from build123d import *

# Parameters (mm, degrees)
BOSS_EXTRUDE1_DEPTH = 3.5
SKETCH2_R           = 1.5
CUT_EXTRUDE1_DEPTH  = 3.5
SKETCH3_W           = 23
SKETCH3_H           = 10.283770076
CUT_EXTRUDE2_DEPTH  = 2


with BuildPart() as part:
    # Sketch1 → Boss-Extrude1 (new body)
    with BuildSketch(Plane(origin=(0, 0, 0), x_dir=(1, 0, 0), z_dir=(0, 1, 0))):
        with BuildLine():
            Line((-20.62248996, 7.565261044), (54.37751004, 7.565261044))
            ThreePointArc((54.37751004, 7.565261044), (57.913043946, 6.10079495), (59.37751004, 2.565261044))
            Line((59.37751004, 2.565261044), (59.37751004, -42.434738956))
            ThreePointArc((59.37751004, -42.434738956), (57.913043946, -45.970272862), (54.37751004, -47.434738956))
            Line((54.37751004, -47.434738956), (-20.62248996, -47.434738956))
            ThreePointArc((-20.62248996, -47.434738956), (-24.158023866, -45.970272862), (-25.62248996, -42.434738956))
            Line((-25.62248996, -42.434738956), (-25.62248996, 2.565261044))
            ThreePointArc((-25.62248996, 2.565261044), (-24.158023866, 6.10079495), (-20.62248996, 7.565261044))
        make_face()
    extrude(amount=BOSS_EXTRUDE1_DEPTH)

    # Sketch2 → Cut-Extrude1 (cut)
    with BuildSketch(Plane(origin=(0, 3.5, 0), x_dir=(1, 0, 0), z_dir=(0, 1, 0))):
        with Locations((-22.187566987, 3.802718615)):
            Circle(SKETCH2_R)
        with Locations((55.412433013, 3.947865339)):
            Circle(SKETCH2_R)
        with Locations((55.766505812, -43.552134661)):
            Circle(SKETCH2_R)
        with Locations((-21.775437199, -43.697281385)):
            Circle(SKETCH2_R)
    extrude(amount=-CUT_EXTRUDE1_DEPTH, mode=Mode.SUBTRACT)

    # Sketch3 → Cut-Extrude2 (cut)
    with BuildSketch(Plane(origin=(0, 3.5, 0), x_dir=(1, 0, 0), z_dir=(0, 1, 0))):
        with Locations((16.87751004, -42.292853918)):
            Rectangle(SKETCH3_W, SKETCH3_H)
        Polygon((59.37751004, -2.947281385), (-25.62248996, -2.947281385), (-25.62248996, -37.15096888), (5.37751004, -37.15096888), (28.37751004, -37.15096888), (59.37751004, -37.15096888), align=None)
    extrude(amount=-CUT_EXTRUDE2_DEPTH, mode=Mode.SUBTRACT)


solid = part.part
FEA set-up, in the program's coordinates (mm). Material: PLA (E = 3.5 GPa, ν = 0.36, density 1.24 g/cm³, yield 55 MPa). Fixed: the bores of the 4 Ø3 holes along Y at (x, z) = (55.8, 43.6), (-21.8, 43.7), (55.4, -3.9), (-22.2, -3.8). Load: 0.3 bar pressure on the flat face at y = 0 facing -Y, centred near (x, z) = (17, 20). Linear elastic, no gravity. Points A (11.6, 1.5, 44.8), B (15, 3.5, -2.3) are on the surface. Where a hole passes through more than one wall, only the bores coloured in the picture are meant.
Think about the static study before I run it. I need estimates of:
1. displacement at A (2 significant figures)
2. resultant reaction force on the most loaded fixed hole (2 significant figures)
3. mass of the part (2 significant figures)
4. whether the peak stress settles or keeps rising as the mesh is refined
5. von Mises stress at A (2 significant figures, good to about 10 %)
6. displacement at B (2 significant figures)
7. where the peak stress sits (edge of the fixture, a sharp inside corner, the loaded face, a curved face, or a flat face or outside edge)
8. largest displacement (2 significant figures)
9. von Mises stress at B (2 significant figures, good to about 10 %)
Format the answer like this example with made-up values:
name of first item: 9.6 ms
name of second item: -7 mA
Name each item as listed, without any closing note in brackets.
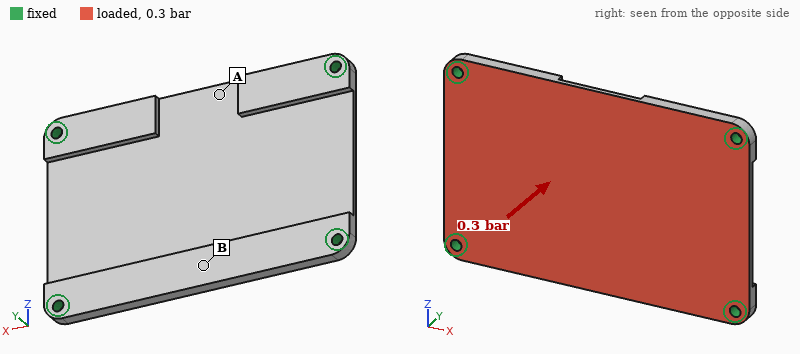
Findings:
displacement at A: 0.63 mm
resultant reaction force on the most loaded fixed hole: 99 N
mass of the part: 12 g
whether the peak stress settles or keeps rising as the mesh is refined: keeps rising
von Mises stress at A: 3.5 MPa
displacement at B: 0.49 mm
where the peak stress sits: edge of the fixture
largest displacement: 0.88 mm
von Mises stress at B: 8.2 MPa
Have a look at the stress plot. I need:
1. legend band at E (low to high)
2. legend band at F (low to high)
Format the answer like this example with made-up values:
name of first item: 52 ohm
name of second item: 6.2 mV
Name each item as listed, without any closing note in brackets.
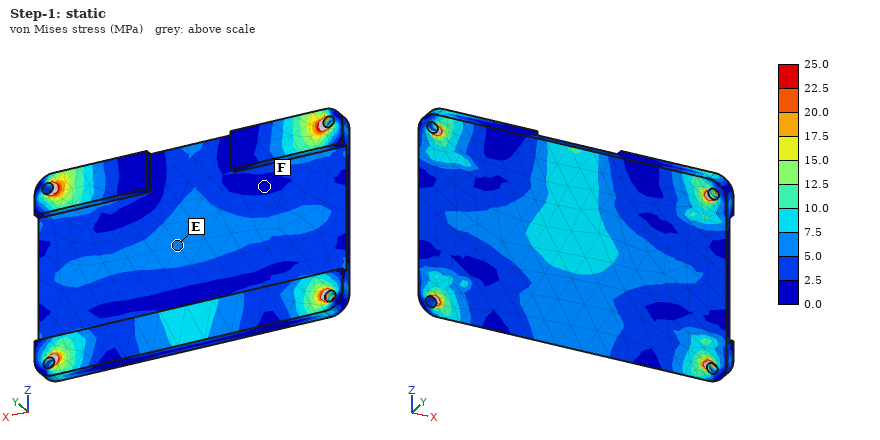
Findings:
legend band at E: 5.0 to 7.5 MPa
legend band at F: 0.0 to 2.5 MPa
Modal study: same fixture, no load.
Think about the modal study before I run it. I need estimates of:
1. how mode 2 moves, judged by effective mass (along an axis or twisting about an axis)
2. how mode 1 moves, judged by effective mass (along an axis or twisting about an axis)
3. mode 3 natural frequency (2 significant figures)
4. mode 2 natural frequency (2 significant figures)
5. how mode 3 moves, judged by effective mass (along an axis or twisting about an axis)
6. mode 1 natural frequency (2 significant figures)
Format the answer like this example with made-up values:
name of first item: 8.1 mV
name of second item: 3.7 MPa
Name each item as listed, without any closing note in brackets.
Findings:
how mode 2 moves, judged by effective mass: twisting about X
how mode 1 moves, judged by effective mass: along Y
mode 3 natural frequency: 1600 Hz
mode 2 natural frequency: 1100 Hz
how mode 3 moves, judged by effective mass: twisting about Z
mode 1 natural frequency: 770 Hz
